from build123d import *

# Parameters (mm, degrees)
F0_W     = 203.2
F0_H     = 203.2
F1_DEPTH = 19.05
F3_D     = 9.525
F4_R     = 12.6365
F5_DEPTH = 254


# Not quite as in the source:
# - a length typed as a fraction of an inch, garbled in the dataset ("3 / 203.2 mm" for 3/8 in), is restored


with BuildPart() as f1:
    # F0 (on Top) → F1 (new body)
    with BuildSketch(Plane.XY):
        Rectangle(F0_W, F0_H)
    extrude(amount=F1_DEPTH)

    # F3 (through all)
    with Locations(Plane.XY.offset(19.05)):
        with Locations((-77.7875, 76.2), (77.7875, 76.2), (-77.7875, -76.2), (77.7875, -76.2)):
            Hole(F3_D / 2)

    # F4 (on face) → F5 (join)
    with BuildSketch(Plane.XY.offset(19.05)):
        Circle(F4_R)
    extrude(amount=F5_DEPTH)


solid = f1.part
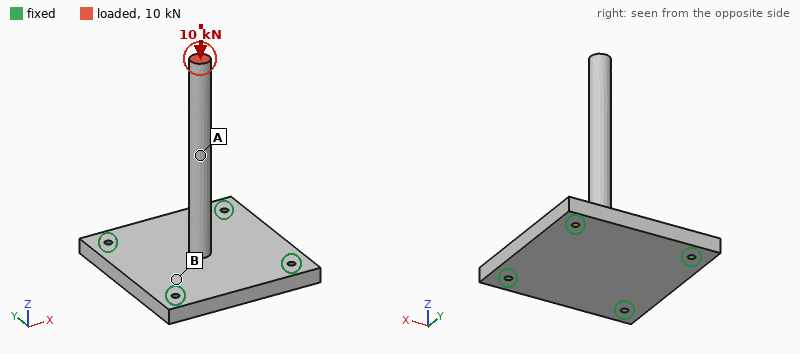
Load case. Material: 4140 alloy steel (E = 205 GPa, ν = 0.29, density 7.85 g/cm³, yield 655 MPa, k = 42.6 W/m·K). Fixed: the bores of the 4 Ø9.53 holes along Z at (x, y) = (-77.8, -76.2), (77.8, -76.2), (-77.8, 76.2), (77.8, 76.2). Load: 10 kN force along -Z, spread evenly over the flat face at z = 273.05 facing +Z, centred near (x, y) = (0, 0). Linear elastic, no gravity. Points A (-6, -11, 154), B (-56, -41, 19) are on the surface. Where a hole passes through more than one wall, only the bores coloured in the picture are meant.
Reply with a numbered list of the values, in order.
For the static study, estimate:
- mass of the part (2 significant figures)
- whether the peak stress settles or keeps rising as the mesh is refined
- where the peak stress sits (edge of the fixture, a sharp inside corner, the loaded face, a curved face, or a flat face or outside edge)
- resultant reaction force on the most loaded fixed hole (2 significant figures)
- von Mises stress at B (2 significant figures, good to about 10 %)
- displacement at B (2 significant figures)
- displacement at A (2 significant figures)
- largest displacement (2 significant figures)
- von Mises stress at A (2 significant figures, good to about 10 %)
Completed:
1. 7.1 kg
2. keeps rising
3. edge of the fixture
4. 2.5 kN
5. 6.0 MPa
6. 11 µm
7. 41 µm
8. 53 µm
9. 20 MPa
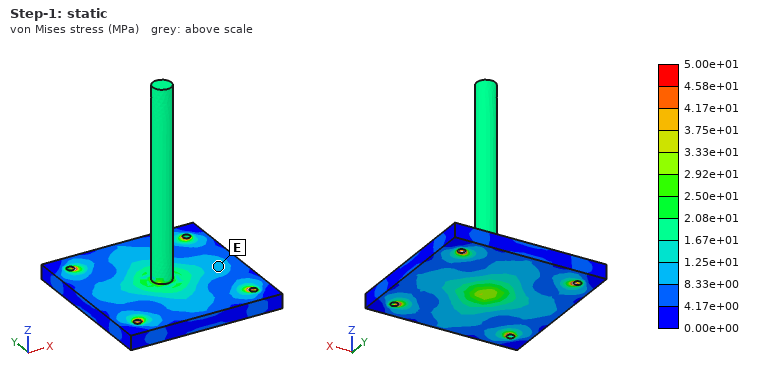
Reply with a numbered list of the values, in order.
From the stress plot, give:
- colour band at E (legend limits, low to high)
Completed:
1. 8.33e+00 to 1.25e+01 MPa
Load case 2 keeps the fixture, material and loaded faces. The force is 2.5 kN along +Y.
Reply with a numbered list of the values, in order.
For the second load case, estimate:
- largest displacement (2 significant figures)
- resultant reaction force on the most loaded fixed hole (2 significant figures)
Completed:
1. 3.7 mm
2. 2.5 kN
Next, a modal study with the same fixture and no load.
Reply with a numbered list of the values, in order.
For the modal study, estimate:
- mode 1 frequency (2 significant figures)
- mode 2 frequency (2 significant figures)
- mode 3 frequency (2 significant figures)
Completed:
1. 260 Hz
2. 260 Hz
3. 1600 Hz
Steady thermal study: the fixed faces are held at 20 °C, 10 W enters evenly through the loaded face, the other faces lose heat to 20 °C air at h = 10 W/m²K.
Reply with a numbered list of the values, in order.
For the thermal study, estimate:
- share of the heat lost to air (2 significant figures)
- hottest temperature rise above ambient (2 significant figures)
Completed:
1. 68 %
2. 71 K
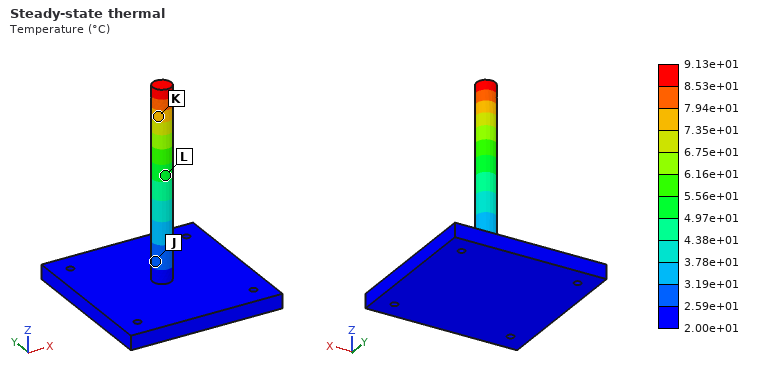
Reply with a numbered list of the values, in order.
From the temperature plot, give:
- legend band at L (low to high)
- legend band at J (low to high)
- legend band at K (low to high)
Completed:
1. 4.97e+01 to 5.56e+01 °C
2. 2.59e+01 to 3.19e+01 °C
3. 7.35e+01 to 7.94e+01 °C
